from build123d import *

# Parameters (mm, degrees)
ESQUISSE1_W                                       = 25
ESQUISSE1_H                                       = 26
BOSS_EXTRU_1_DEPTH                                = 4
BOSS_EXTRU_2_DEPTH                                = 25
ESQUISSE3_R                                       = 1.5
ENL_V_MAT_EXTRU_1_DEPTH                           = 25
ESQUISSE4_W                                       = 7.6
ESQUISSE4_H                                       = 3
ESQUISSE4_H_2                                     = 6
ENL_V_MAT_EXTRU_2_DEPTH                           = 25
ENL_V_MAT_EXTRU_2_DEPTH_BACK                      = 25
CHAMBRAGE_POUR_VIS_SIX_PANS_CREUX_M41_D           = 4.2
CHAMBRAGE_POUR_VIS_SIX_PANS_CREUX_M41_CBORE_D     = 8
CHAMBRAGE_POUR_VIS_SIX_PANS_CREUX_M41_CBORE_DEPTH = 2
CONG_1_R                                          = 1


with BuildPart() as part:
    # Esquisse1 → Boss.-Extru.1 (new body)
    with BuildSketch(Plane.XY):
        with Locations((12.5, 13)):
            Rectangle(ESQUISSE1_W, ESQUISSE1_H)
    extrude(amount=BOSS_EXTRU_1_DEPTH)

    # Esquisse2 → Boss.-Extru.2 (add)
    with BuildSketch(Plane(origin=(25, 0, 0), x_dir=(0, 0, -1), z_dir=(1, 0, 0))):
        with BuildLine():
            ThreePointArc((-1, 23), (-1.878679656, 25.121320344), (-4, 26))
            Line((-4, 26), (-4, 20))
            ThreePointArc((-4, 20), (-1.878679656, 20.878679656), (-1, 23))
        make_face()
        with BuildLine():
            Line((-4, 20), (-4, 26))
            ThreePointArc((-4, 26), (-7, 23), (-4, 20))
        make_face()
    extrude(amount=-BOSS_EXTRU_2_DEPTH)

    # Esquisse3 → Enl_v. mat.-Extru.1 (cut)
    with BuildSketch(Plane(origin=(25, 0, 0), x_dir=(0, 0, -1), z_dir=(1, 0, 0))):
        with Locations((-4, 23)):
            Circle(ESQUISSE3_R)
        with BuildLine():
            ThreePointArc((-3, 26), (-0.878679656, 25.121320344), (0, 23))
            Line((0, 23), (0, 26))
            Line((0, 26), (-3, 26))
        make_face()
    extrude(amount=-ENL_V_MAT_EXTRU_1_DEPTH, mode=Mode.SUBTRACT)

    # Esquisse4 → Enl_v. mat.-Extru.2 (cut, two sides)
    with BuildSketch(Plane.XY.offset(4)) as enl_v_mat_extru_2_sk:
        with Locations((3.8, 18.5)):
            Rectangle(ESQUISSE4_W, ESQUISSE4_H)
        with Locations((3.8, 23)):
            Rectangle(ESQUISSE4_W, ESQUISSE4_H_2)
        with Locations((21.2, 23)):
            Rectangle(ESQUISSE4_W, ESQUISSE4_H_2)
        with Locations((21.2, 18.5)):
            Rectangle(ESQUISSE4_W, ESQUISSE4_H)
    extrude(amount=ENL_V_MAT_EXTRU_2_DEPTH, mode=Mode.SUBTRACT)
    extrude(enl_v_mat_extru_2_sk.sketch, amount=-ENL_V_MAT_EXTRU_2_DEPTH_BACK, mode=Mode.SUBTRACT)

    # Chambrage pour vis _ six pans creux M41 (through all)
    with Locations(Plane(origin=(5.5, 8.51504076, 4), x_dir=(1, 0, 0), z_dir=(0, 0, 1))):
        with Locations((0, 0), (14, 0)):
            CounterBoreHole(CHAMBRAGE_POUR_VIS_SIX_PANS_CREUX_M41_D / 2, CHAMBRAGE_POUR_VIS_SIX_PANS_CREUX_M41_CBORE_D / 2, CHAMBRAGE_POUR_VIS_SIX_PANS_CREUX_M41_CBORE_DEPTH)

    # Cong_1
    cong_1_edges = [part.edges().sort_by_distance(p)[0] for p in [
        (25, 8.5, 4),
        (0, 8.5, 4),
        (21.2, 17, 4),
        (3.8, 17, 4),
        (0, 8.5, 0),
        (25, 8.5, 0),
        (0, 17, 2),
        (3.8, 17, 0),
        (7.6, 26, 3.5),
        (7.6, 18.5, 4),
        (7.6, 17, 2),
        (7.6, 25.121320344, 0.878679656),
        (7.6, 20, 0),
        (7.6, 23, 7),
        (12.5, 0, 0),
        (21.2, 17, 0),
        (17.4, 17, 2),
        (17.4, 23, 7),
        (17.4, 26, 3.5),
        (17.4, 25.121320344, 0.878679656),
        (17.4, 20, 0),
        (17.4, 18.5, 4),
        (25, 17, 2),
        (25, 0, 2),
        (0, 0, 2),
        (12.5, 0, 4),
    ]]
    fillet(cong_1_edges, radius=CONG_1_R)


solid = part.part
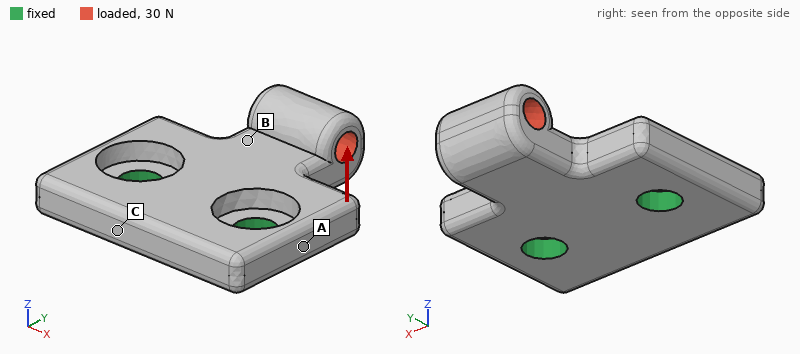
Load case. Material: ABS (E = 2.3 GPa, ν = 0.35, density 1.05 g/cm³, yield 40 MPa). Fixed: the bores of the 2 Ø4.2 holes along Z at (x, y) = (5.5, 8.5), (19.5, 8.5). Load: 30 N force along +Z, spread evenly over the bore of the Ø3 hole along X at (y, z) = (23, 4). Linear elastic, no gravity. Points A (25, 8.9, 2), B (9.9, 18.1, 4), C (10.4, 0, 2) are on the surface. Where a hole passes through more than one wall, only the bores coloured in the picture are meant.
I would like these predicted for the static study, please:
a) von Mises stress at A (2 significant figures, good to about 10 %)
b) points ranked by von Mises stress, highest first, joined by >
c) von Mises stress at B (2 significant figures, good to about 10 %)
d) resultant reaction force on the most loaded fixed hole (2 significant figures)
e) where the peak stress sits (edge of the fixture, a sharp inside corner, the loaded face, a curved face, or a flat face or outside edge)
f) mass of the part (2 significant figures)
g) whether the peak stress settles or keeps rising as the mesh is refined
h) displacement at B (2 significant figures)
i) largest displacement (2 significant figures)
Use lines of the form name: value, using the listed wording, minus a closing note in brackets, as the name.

von Mises stress at A: 3.4 MPa
points ranked by von Mises stress, highest first, joined by >: B > A > C
von Mises stress at B: 6.3 MPa
resultant reaction force on the most loaded fixed hole: 20 N
where the peak stress sits: edge of the fixture
mass of the part: 1.9 g
whether the peak stress settles or keeps rising as the mesh is refined: keeps rising
displacement at B: 0.14 mm
largest displacement: 0.33 mm
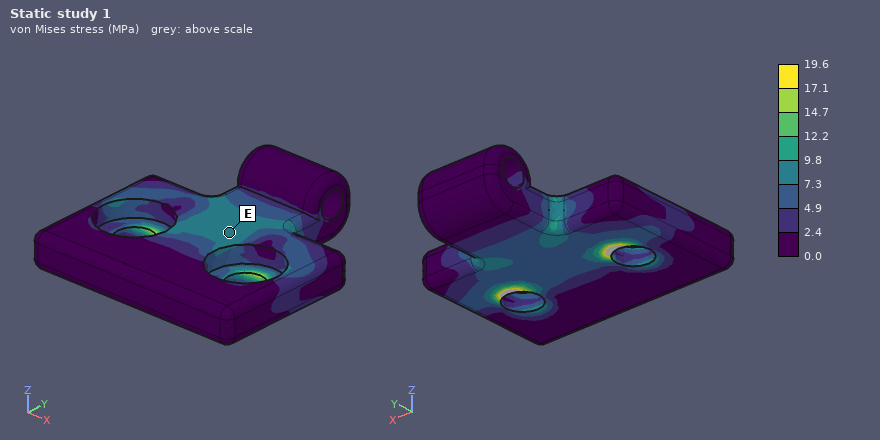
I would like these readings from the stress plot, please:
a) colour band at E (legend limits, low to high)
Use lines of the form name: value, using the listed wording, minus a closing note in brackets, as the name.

colour band at E: 7.3 to 9.8 MPa
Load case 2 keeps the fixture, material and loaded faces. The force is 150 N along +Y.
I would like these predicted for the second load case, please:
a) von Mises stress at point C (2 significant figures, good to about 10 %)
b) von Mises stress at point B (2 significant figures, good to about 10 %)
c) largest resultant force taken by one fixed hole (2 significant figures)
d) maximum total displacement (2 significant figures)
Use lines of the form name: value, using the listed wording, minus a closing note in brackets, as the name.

von Mises stress at point C: 1.6 MPa
von Mises stress at point B: 14 MPa
largest resultant force taken by one fixed hole: 76 N
maximum total displacement: 0.44 mm
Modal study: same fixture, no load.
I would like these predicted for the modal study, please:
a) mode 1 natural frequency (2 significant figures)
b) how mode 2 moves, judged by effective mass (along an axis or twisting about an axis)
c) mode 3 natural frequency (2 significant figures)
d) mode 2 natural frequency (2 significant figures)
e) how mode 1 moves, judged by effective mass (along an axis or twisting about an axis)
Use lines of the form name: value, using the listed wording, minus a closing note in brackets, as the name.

mode 1 natural frequency: 2800 Hz
how mode 2 moves, judged by effective mass: along Z
mode 3 natural frequency: 8800 Hz
mode 2 natural frequency: 8200 Hz
how mode 1 moves, judged by effective mass: along Z
